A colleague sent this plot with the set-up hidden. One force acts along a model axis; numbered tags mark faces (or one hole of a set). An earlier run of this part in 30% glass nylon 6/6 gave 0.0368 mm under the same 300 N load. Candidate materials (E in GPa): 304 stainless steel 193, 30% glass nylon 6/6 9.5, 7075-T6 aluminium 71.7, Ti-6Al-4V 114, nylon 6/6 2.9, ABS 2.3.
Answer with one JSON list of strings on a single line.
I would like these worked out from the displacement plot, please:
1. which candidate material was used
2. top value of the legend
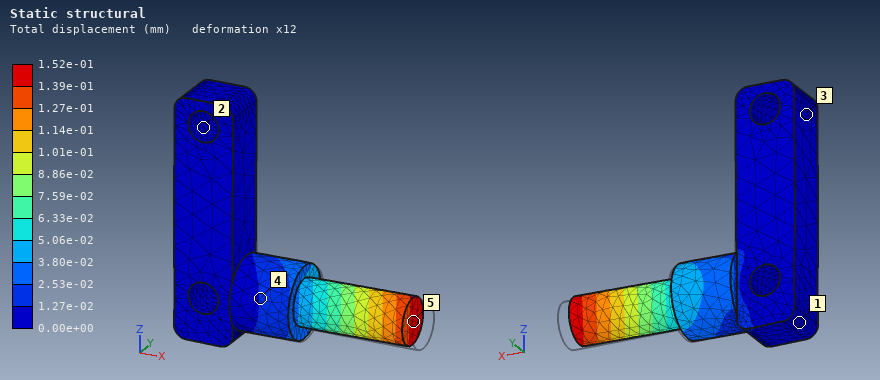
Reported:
["ABS", "1.52e-01 mm"]
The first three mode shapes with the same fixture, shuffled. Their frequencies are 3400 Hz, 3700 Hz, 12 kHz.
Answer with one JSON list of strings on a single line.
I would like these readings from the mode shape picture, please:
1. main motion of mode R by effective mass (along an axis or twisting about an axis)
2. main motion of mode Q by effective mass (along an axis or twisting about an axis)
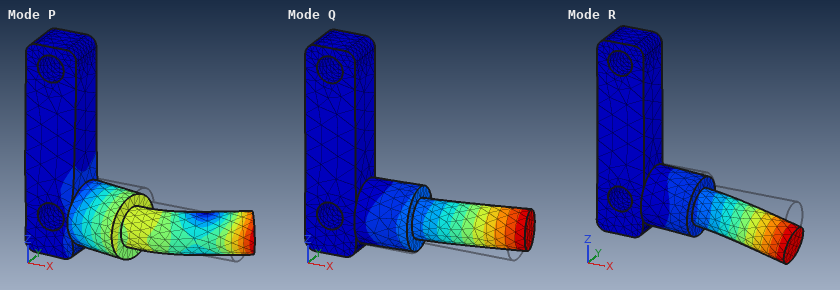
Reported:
["along Z", "along Y"]
